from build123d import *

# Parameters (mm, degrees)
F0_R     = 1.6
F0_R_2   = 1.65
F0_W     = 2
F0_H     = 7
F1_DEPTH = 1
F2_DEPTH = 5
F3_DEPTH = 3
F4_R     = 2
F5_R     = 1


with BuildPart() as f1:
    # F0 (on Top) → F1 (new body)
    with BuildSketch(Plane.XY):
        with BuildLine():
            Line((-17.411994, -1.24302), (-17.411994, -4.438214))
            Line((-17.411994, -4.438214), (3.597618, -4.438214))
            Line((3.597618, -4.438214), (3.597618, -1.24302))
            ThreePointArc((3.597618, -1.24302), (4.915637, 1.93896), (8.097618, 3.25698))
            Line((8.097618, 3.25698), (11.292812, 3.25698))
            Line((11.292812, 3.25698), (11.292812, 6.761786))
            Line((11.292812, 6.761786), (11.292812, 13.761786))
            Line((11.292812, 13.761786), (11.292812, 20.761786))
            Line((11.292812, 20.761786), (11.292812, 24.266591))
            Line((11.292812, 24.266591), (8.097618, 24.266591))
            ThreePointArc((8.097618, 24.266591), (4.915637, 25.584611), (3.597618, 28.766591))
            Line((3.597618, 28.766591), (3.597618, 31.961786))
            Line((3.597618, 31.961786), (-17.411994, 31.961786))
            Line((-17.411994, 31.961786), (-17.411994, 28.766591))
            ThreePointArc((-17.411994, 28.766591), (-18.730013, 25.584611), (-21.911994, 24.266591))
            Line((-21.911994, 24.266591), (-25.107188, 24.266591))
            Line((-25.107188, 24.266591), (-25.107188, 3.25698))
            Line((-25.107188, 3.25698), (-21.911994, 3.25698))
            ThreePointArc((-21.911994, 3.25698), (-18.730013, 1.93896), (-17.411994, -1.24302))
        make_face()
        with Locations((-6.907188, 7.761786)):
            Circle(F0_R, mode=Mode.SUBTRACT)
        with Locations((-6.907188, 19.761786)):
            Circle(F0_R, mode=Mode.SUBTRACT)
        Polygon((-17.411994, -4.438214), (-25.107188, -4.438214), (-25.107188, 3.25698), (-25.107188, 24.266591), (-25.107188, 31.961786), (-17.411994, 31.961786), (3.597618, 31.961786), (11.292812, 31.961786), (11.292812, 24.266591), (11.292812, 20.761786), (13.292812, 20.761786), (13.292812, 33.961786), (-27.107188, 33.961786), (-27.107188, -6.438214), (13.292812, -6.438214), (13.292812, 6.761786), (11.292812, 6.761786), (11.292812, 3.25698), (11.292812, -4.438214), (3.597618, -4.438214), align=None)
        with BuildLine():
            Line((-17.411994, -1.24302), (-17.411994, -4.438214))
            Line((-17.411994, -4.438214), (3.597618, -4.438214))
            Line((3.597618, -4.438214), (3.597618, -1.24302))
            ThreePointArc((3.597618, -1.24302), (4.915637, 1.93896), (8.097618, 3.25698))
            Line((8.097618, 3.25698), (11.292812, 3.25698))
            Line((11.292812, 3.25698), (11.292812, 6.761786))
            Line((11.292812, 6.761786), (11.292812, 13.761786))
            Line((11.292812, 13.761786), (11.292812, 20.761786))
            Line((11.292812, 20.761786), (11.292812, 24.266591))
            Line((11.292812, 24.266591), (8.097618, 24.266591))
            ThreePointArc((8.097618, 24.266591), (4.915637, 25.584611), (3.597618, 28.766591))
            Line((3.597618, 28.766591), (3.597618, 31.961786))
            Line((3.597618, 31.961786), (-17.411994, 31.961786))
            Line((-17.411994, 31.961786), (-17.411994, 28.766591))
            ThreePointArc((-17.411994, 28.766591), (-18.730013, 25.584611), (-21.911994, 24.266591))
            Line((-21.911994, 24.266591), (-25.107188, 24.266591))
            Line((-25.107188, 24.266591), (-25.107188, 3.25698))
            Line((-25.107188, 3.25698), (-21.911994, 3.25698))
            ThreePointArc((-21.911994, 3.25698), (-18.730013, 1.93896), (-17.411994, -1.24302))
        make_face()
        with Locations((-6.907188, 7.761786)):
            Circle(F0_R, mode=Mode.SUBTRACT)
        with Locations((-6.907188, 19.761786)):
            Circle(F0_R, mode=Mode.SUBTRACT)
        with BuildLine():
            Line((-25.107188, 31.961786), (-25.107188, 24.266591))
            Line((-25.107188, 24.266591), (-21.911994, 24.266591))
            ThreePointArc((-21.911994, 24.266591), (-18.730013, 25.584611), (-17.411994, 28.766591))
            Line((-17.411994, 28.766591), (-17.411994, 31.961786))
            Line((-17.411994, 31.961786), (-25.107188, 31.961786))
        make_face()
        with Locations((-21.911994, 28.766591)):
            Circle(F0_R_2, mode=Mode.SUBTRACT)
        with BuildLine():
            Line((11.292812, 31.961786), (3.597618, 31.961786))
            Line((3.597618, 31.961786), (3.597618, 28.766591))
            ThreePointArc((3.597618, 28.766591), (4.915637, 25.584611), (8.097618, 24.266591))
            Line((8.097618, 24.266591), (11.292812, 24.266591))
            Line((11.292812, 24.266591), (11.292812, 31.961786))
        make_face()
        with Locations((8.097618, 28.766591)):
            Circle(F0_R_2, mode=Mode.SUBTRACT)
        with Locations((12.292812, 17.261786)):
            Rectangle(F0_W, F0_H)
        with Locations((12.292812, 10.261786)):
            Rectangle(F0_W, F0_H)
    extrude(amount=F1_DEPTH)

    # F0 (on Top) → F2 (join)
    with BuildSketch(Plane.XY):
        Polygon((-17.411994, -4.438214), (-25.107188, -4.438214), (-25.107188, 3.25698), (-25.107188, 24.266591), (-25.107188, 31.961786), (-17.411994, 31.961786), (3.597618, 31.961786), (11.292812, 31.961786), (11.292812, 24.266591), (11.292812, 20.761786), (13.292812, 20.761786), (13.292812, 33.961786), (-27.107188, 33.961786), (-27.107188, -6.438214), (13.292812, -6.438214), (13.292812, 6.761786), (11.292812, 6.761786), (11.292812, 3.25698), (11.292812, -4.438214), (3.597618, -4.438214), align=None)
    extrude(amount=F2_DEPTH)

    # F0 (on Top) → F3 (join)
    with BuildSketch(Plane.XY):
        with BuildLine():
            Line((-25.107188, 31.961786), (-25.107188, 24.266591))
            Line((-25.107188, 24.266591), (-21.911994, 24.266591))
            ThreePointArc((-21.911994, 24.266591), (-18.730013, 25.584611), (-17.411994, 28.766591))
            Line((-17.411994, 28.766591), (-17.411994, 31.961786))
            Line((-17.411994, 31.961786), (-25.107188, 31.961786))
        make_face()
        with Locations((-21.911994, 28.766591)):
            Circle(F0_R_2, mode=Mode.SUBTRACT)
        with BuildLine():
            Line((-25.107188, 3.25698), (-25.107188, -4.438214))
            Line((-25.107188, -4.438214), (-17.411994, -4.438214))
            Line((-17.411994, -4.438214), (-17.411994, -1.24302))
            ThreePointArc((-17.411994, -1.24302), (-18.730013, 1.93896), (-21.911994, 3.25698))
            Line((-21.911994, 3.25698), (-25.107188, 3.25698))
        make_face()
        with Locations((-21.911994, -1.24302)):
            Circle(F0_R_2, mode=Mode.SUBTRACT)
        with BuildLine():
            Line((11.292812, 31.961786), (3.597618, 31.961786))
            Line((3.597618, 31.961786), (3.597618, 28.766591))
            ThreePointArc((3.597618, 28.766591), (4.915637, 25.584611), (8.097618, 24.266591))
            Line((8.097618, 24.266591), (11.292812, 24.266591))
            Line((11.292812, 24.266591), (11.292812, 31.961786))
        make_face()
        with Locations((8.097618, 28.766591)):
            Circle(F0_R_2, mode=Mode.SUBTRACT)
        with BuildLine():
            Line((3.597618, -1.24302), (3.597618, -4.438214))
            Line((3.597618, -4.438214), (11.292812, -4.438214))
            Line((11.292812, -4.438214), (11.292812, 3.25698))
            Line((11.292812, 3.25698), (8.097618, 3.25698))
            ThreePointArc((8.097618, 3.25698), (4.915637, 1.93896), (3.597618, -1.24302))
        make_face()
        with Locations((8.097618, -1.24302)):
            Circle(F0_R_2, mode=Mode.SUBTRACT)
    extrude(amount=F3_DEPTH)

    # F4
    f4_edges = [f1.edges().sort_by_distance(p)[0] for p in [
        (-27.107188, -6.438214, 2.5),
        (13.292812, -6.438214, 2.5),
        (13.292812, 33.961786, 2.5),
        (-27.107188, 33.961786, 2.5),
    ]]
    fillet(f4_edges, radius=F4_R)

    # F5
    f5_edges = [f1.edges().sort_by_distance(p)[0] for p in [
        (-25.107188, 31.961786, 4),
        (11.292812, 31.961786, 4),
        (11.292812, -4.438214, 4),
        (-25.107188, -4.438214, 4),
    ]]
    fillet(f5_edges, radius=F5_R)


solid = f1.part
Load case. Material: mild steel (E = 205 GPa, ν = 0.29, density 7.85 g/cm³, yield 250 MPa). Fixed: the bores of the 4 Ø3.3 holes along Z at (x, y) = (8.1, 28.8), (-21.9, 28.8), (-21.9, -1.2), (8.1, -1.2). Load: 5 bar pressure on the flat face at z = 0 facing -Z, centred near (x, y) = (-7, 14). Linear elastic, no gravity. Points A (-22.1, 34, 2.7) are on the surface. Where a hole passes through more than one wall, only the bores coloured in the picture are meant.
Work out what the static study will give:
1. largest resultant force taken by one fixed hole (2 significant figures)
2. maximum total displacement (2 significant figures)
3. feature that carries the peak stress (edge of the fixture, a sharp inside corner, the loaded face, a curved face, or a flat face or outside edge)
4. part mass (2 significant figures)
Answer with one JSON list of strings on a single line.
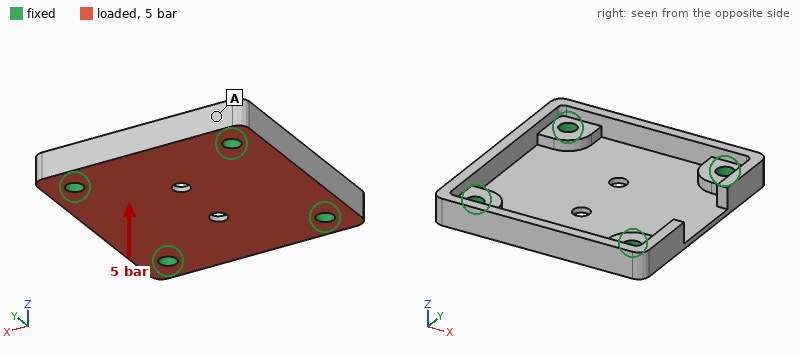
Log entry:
["220 N", "58 µm", "the loaded face", "24 g"]
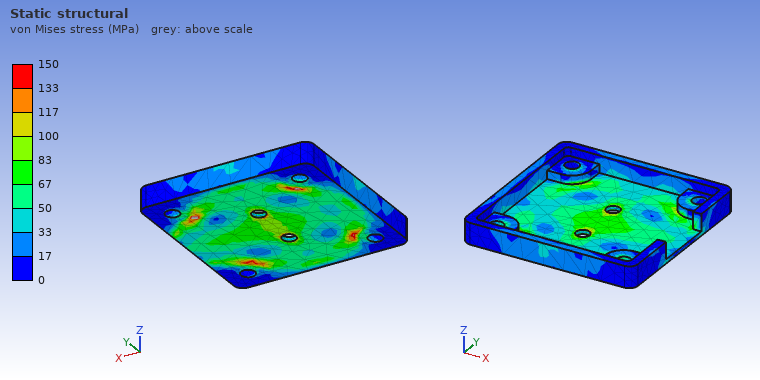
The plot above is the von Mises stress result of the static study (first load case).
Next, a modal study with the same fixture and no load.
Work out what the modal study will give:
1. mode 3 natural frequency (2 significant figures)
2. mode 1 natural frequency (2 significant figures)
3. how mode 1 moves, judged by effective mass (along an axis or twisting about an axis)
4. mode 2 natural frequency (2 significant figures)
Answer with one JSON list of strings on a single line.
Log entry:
["14 kHz", "6800 Hz", "along Z", "13 kHz"]
